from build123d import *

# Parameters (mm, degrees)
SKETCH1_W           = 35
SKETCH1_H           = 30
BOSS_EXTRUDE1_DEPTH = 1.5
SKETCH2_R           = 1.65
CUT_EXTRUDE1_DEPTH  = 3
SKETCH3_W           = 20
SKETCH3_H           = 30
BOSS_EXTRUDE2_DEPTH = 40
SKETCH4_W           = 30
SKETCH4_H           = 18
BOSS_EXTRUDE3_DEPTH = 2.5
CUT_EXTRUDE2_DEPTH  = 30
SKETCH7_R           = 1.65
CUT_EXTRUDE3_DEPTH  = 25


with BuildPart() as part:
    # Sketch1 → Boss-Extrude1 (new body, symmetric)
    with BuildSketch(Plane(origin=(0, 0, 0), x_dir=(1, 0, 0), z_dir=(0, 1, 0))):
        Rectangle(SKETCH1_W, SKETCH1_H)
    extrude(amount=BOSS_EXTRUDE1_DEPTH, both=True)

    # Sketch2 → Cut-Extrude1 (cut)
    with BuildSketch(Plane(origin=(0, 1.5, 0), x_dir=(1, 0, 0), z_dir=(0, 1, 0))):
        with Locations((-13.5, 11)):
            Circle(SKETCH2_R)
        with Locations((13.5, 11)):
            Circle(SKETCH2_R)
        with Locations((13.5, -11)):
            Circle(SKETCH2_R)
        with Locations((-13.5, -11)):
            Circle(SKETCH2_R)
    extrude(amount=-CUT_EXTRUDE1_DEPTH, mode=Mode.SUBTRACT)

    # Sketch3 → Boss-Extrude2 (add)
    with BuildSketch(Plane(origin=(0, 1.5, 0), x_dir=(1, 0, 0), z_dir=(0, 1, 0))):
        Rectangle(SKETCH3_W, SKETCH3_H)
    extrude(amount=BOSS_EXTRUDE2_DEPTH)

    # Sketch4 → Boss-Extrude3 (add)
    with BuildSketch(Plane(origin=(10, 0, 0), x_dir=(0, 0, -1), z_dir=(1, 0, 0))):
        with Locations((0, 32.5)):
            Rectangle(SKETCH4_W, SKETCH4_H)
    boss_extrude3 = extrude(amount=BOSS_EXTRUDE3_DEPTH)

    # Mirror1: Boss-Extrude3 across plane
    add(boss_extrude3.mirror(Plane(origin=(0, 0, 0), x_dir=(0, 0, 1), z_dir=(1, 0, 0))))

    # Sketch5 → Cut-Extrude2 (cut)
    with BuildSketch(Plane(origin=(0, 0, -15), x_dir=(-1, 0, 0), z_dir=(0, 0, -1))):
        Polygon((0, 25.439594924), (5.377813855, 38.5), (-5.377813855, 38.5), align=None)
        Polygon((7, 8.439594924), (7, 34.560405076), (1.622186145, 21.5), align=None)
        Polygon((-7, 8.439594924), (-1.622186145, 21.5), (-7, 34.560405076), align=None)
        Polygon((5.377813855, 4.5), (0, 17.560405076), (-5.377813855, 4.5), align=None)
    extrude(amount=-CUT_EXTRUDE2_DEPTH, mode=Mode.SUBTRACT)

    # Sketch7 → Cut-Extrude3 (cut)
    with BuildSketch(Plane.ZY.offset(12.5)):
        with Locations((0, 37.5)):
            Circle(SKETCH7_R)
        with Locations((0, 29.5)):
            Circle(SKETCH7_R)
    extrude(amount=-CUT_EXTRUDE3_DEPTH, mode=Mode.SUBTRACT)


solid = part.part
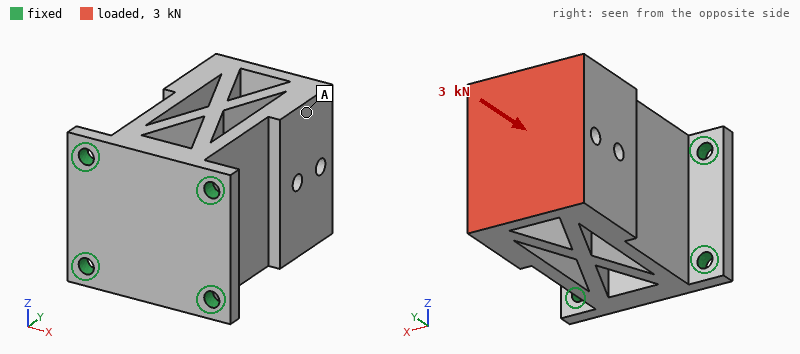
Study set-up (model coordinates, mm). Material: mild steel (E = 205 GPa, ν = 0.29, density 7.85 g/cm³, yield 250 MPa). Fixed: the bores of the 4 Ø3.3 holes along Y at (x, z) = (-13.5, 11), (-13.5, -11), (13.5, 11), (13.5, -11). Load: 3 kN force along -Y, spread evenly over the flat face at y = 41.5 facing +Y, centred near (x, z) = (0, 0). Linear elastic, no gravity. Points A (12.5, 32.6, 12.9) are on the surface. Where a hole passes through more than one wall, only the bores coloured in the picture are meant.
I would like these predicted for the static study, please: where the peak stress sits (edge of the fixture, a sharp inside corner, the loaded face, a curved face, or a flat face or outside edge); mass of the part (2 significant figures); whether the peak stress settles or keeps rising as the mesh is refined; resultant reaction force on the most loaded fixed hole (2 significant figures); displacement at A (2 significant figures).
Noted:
edge of the fixture
170 g
keeps rising
810 N
4.2 µm
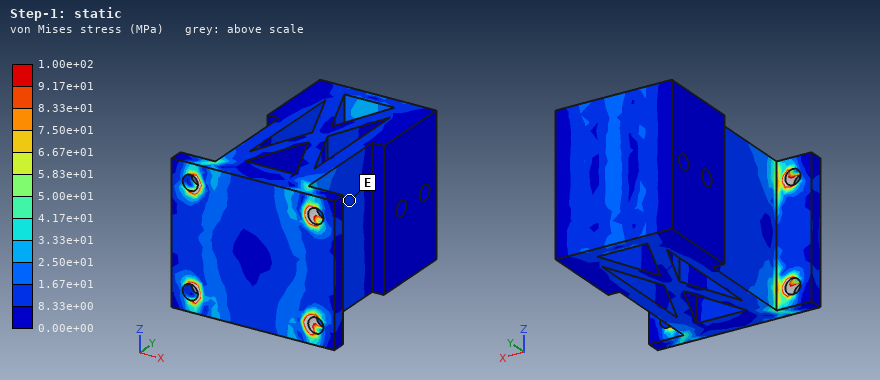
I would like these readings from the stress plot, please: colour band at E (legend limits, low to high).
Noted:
8.33e+00 to 1.67e+01 MPa
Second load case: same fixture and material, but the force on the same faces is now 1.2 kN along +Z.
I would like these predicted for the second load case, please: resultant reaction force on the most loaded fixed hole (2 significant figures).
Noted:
1.2 kN
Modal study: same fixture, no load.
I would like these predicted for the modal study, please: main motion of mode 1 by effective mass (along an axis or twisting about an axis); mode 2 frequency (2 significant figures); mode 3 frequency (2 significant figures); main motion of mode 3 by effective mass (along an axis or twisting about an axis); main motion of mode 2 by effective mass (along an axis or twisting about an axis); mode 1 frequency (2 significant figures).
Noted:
along X
4700 Hz
9400 Hz
twisting about Y
along Z
4400 Hz
